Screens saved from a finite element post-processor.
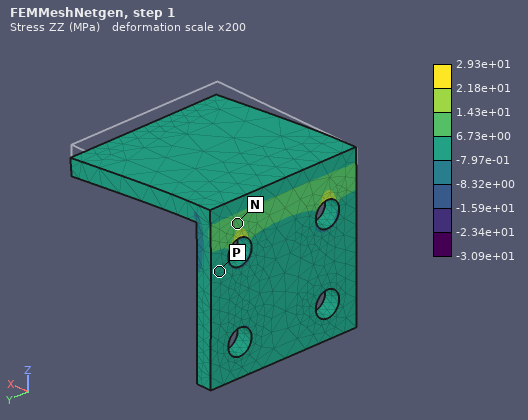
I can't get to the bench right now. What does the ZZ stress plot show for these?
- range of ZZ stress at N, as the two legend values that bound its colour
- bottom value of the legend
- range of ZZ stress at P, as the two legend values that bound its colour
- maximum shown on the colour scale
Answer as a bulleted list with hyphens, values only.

- 6.73e+00 to 1.43e+01 MPa
- -3.09e+01 MPa
- -7.97e-01 to 6.73e+00 MPa
- 2.93e+01 MPa
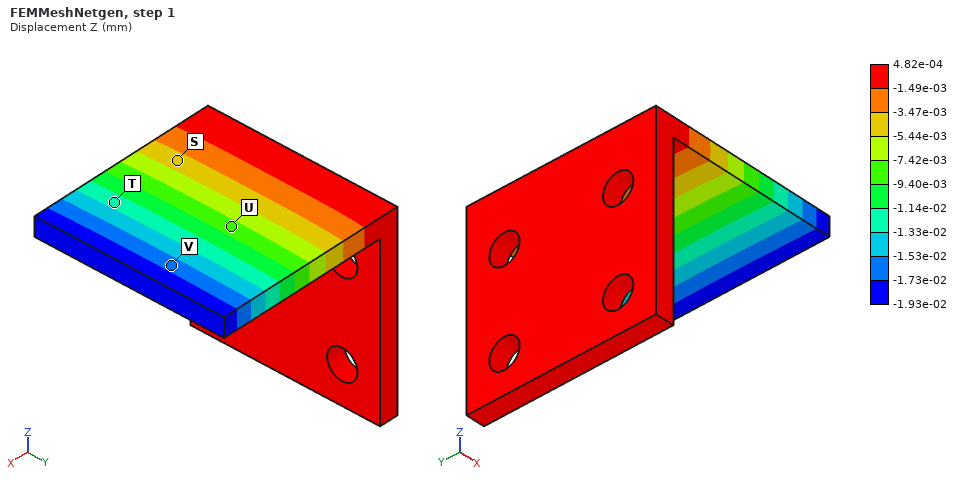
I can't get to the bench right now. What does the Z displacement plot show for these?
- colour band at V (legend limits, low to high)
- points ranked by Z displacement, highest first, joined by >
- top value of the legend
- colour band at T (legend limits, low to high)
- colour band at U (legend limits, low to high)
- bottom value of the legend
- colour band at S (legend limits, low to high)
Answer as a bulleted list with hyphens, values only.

- -1.73e-02 to -1.53e-02 mm
- S > U > T > V
- 4.82e-04 mm
- -1.33e-02 to -1.14e-02 mm
- -9.40e-03 to -7.42e-03 mm
- -1.93e-02 mm
- -5.44e-03 to -3.47e-03 mm
